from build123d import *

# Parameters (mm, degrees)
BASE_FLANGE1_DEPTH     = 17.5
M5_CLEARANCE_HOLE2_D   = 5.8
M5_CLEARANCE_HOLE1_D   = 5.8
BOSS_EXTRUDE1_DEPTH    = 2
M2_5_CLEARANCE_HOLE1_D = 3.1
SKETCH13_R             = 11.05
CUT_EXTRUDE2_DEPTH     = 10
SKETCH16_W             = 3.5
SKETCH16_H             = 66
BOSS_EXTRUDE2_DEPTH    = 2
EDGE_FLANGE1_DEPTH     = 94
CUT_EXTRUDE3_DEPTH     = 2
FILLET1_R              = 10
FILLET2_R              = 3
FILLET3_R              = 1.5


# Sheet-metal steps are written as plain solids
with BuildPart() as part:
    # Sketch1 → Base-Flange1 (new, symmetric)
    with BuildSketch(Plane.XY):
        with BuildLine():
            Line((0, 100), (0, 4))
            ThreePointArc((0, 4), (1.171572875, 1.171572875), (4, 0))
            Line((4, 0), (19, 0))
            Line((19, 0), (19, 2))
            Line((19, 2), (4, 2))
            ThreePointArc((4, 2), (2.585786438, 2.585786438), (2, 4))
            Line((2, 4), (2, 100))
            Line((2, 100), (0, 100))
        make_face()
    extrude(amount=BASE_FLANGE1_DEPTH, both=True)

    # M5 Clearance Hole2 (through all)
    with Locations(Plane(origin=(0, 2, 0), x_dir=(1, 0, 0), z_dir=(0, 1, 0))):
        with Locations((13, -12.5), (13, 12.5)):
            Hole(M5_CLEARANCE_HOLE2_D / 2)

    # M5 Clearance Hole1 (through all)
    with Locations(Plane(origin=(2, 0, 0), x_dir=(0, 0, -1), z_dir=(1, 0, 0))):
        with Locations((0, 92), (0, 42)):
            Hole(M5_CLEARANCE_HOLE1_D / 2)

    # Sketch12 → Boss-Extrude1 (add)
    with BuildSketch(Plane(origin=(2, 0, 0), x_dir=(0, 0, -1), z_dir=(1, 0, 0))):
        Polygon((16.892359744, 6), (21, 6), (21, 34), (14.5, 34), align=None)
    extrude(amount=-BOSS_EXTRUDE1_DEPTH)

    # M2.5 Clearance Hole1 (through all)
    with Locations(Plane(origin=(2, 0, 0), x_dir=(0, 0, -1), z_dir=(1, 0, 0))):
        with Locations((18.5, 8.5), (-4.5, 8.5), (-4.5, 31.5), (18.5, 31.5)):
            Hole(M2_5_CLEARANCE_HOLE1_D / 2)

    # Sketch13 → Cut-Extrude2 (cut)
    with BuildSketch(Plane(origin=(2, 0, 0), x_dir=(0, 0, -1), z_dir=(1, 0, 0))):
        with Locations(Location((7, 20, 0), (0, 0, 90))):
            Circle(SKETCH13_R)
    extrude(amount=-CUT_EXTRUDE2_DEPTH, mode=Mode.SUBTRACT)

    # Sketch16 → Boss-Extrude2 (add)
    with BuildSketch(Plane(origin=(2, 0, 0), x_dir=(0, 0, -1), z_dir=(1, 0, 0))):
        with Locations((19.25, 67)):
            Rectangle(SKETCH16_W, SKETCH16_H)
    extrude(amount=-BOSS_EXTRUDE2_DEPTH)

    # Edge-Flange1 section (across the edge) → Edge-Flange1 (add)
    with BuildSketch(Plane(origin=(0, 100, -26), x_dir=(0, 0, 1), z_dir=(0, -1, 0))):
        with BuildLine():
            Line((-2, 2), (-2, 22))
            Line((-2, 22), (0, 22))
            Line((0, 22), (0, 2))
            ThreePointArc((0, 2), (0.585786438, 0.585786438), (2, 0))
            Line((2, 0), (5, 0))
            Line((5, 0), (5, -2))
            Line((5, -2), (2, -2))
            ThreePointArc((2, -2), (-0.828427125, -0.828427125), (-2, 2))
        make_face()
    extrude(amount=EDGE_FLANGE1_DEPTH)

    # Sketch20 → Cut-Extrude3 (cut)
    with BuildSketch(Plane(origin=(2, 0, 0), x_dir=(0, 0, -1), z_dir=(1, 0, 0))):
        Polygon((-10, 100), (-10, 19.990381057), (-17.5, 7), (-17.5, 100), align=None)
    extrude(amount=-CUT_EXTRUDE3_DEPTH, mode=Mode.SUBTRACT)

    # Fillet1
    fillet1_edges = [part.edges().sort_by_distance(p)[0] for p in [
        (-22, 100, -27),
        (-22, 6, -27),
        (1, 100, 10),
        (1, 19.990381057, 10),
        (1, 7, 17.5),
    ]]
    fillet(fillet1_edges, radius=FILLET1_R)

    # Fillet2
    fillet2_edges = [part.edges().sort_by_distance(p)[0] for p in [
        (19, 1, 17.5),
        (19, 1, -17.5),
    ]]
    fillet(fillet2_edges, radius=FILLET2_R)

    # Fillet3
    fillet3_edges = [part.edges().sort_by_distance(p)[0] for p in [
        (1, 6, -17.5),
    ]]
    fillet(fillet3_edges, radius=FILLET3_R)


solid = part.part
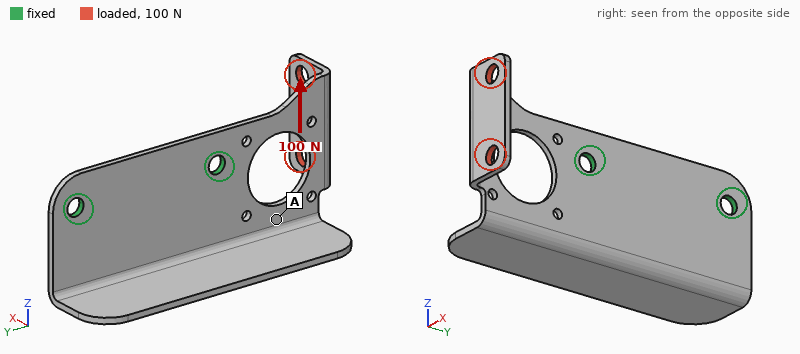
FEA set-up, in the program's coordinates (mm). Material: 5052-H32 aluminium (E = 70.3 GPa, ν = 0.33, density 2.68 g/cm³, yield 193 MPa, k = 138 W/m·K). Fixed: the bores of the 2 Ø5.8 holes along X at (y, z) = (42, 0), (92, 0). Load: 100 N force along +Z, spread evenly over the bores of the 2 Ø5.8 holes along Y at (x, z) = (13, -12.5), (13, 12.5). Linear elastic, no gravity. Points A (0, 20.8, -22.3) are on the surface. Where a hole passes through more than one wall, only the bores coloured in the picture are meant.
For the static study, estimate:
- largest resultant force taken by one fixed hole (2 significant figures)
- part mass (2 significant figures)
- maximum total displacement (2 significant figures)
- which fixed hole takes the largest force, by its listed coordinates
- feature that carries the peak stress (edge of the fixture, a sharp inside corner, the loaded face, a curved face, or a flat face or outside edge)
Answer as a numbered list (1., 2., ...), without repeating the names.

1. 180 N
2. 31 g
3. 0.84 mm
4. (42, 0)
5. a curved face
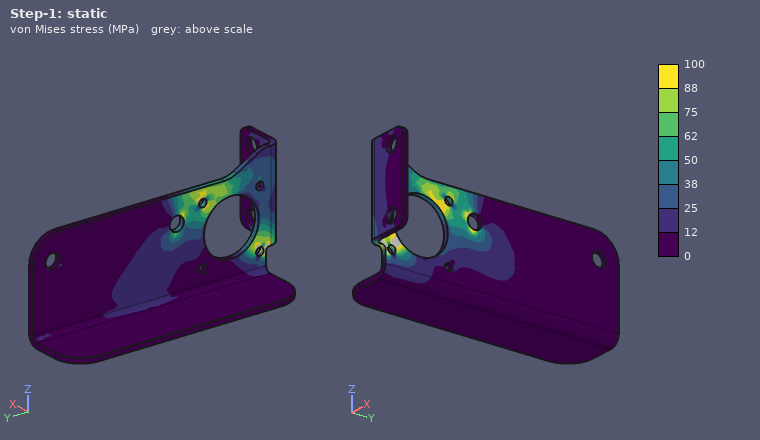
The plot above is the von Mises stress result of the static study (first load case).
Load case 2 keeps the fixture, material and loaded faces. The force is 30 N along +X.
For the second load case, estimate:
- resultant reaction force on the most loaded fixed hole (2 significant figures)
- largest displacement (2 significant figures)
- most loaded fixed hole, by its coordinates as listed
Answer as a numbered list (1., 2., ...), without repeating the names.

1. 44 N
2. 0.54 mm
3. (42, 0)
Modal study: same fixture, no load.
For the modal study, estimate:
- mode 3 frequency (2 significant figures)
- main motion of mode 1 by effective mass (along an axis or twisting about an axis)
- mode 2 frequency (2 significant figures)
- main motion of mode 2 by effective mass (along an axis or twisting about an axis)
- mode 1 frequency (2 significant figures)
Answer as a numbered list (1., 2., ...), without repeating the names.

1. 1200 Hz
2. along X
3. 740 Hz
4. along X
5. 650 Hz
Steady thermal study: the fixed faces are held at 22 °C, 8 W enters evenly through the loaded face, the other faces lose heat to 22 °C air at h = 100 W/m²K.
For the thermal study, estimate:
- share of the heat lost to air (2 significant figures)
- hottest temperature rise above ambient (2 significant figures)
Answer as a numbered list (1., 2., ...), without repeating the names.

1. 79 %
2. 32 K
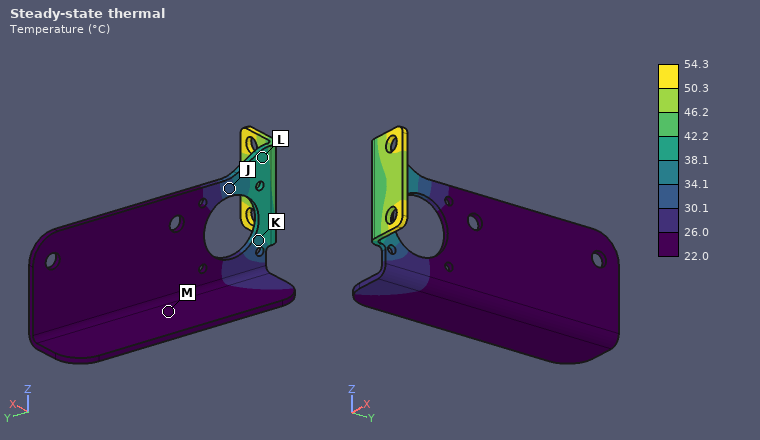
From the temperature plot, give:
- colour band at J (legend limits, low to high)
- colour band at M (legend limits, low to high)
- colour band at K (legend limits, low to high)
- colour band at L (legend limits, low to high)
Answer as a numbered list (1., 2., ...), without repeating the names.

1. 30.1 to 34.1 °C
2. 22.0 to 26.0 °C
3. 34.1 to 38.1 °C
4. 38.1 to 42.2 °C
